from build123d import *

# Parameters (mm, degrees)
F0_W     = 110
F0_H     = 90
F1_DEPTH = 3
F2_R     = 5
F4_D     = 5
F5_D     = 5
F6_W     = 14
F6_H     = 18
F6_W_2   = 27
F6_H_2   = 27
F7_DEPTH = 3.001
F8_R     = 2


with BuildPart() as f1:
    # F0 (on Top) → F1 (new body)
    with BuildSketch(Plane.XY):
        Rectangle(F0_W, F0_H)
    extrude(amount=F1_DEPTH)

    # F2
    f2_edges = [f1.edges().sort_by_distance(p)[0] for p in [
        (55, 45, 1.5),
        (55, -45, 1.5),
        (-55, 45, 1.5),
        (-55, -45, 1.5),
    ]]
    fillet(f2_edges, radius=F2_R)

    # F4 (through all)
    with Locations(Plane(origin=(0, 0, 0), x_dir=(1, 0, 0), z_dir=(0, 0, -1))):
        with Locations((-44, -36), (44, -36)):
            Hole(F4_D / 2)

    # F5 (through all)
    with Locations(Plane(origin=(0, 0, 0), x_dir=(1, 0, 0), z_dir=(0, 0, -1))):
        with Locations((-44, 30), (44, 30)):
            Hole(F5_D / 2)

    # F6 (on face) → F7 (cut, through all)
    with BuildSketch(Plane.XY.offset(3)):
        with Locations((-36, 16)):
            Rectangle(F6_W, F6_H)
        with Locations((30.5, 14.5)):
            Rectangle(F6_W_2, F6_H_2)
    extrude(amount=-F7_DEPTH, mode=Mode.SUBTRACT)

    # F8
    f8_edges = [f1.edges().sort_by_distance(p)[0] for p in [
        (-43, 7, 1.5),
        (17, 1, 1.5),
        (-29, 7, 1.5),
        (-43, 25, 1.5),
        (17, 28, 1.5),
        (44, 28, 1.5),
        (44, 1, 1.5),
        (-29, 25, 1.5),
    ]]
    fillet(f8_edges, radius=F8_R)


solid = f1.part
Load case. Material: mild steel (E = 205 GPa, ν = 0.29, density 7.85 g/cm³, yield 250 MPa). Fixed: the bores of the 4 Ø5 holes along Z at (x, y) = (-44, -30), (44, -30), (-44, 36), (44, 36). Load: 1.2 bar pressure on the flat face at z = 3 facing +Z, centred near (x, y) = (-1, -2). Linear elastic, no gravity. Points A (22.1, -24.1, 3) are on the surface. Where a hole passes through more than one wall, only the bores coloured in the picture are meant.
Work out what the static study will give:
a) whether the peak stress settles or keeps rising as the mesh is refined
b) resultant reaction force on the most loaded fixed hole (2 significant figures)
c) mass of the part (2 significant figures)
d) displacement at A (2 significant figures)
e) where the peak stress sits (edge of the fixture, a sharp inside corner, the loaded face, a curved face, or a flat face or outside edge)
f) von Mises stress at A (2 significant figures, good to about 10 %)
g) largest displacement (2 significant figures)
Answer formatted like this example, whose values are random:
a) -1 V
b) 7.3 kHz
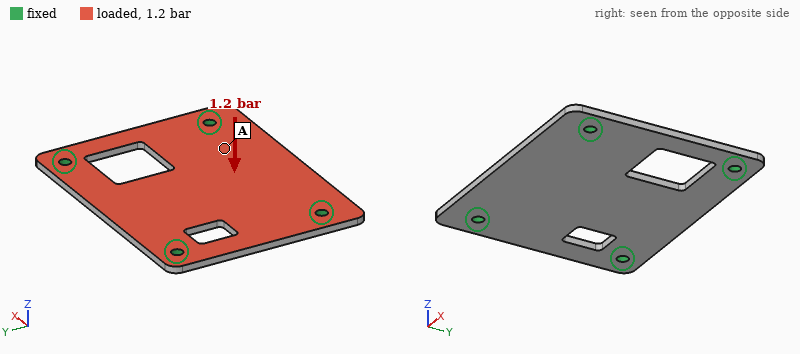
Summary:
a) keeps rising
b) 310 N
c) 210 g
d) 33 µm
e) edge of the fixture
f) 14 MPa
g) 65 µm
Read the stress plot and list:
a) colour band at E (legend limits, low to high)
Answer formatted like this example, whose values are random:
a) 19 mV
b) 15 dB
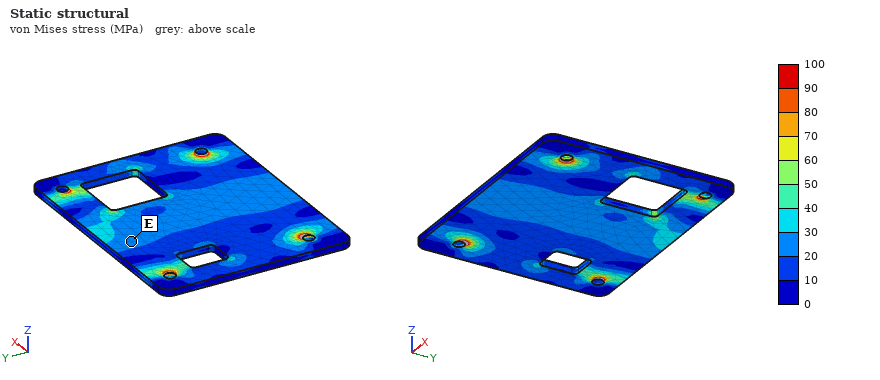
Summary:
a) 20 to 30 MPa
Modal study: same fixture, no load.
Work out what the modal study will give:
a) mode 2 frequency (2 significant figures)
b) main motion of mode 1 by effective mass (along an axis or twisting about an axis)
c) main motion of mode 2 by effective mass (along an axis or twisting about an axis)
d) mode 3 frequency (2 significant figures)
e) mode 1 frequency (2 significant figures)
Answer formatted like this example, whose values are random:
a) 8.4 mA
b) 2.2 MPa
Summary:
a) 2300 Hz
b) along Z
c) twisting about X
d) 3100 Hz
e) 1700 Hz
